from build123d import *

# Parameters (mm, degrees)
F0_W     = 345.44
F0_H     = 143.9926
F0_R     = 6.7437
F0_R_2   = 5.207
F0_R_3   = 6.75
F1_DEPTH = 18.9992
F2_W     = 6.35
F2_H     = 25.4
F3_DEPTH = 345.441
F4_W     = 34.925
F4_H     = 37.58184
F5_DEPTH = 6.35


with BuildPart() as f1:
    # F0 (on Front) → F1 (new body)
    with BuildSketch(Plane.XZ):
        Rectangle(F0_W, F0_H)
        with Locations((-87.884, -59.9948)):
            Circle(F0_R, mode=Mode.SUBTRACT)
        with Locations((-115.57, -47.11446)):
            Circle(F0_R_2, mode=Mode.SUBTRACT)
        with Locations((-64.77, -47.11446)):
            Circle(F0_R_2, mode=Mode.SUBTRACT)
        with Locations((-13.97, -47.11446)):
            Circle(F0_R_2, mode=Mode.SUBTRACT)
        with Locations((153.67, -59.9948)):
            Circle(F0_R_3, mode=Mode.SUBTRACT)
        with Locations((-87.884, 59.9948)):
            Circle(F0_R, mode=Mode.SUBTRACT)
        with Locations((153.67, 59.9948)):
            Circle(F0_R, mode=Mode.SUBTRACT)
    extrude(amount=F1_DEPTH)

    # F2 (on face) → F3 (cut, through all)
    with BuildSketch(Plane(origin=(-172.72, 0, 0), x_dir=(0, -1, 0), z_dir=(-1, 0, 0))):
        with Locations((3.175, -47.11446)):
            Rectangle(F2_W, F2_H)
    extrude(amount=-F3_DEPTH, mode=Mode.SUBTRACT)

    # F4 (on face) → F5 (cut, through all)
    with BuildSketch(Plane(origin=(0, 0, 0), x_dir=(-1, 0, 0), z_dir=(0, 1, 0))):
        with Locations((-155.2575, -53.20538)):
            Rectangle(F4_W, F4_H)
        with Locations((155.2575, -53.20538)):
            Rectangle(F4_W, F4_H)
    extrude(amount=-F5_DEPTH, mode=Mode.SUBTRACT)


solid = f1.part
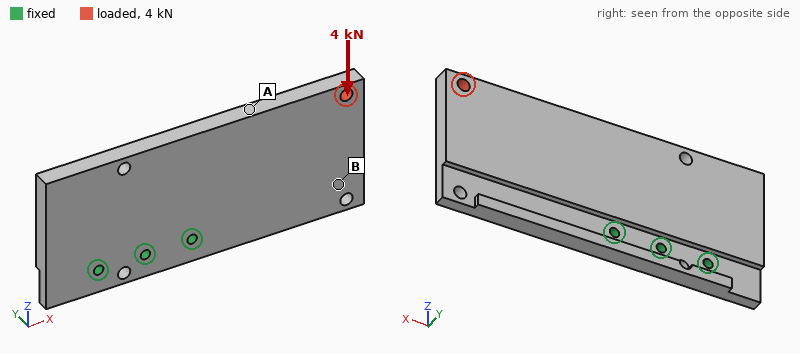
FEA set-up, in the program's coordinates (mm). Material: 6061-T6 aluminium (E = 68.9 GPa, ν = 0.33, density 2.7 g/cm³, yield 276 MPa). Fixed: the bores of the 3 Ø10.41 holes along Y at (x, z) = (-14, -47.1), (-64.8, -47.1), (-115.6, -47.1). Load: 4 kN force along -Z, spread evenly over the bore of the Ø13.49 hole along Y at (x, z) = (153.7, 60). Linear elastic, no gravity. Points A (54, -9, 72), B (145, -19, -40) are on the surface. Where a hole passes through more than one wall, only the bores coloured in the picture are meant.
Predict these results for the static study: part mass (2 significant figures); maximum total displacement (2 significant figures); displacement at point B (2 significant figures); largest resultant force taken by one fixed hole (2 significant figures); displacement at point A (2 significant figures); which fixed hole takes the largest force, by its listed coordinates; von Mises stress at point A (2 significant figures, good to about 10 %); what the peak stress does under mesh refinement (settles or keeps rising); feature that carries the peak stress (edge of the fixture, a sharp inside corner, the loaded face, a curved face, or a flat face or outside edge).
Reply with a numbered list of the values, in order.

1. 2.4 kg
2. 0.13 mm
3. 0.084 mm
4. 10 kN
5. 0.068 mm
6. (-14, -47.1)
7. 7.3 MPa
8. keeps rising
9. edge of the fixture
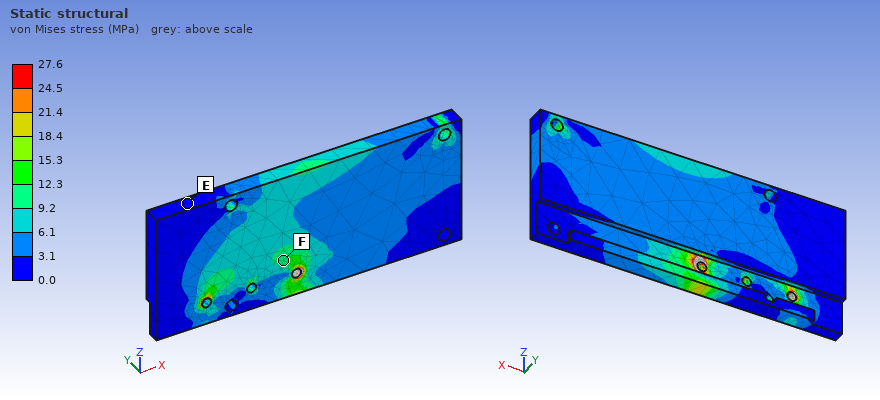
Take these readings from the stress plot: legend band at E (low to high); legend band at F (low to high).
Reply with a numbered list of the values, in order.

1. 0.0 to 3.1 MPa
2. 9.2 to 12.3 MPa
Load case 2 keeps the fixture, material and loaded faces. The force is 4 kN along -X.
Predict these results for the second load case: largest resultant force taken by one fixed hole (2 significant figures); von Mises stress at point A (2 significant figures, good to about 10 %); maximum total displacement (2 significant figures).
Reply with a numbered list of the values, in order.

1. 4.2 kN
2. 5.7 MPa
3. 59 µm
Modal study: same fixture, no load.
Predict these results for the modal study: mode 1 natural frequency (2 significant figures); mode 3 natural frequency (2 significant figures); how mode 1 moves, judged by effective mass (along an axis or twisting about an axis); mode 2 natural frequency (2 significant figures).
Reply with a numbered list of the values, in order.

1. 310 Hz
2. 1000 Hz
3. along Y
4. 620 Hz
